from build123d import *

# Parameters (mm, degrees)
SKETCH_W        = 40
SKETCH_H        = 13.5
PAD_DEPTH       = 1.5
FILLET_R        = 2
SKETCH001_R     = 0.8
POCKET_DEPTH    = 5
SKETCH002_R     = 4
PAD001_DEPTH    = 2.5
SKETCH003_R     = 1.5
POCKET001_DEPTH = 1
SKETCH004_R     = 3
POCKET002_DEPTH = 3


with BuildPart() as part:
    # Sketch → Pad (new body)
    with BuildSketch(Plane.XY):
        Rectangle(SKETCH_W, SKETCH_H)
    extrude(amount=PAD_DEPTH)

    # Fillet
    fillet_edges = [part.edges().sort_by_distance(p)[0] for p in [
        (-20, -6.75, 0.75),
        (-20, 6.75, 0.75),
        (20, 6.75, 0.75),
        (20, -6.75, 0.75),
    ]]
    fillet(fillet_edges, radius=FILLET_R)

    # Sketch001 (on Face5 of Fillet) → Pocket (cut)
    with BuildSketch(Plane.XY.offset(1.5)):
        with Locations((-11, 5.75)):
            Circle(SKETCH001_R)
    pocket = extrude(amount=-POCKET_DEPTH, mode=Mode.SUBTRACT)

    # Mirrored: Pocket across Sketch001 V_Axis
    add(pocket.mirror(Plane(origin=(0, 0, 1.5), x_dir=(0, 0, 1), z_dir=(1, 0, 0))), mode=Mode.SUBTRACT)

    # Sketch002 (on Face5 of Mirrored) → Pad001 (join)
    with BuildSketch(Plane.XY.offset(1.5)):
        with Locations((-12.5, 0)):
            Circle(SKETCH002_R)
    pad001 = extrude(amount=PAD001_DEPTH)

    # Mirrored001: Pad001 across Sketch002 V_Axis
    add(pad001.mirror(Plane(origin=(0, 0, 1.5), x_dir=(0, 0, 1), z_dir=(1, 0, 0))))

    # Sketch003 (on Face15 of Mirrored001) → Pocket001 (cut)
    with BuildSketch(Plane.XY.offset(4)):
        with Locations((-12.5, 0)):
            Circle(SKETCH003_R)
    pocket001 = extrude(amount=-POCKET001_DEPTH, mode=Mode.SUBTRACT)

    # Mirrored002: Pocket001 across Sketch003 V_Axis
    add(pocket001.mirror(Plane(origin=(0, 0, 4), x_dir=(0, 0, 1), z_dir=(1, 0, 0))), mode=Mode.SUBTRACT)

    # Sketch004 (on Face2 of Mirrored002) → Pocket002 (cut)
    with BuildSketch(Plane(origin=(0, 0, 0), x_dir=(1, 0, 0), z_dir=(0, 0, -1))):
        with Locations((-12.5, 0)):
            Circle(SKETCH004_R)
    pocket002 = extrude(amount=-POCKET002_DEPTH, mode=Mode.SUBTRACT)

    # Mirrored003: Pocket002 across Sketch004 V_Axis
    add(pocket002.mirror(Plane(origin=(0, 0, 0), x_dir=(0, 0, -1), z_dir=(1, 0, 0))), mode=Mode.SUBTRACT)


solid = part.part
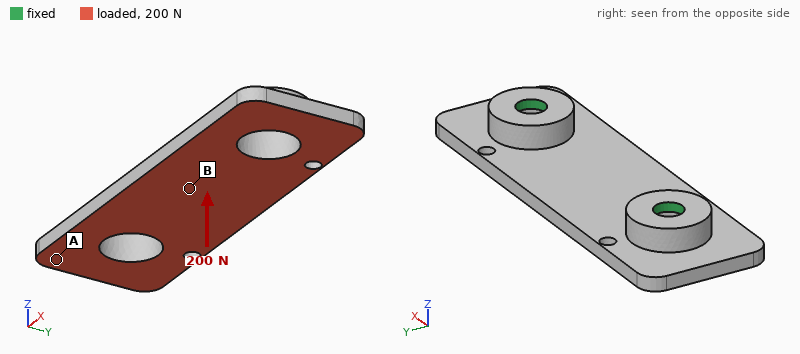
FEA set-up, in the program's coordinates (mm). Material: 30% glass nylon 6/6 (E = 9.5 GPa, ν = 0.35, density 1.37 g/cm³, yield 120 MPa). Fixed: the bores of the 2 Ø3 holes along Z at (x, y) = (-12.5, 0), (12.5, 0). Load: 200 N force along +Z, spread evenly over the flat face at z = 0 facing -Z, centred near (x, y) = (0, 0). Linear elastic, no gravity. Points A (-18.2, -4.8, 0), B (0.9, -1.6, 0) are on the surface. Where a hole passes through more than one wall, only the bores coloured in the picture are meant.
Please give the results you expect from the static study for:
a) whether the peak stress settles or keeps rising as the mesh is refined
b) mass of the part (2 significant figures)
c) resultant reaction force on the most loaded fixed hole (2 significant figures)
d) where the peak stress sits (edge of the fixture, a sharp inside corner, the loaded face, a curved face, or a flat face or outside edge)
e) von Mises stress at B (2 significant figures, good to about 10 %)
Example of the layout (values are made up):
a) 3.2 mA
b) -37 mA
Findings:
a) keeps rising
b) 1.2 g
c) 110 N
d) edge of the fixture
e) 23 MPa
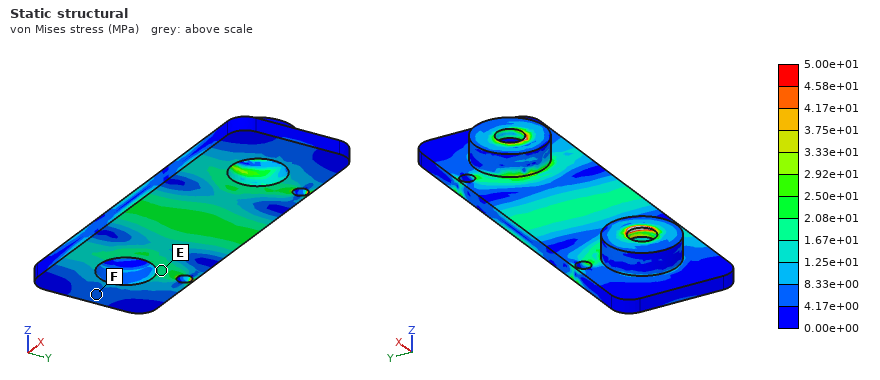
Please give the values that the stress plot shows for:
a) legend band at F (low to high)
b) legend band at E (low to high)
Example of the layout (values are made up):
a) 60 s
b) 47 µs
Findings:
a) 4.17e+00 to 8.33e+00 MPa
b) 1.67e+01 to 2.08e+01 MPa
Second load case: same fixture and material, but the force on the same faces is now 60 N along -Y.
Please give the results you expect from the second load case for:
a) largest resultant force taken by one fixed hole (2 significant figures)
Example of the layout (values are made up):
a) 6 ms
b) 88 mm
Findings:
a) 30 N
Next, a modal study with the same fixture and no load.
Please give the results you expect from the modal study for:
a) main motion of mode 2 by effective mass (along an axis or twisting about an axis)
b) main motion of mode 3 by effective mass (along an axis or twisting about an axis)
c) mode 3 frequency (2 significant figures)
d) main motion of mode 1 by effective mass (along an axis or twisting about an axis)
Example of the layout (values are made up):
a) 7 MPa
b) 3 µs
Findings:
a) along Z
b) along X
c) 9500 Hz
d) along Y
